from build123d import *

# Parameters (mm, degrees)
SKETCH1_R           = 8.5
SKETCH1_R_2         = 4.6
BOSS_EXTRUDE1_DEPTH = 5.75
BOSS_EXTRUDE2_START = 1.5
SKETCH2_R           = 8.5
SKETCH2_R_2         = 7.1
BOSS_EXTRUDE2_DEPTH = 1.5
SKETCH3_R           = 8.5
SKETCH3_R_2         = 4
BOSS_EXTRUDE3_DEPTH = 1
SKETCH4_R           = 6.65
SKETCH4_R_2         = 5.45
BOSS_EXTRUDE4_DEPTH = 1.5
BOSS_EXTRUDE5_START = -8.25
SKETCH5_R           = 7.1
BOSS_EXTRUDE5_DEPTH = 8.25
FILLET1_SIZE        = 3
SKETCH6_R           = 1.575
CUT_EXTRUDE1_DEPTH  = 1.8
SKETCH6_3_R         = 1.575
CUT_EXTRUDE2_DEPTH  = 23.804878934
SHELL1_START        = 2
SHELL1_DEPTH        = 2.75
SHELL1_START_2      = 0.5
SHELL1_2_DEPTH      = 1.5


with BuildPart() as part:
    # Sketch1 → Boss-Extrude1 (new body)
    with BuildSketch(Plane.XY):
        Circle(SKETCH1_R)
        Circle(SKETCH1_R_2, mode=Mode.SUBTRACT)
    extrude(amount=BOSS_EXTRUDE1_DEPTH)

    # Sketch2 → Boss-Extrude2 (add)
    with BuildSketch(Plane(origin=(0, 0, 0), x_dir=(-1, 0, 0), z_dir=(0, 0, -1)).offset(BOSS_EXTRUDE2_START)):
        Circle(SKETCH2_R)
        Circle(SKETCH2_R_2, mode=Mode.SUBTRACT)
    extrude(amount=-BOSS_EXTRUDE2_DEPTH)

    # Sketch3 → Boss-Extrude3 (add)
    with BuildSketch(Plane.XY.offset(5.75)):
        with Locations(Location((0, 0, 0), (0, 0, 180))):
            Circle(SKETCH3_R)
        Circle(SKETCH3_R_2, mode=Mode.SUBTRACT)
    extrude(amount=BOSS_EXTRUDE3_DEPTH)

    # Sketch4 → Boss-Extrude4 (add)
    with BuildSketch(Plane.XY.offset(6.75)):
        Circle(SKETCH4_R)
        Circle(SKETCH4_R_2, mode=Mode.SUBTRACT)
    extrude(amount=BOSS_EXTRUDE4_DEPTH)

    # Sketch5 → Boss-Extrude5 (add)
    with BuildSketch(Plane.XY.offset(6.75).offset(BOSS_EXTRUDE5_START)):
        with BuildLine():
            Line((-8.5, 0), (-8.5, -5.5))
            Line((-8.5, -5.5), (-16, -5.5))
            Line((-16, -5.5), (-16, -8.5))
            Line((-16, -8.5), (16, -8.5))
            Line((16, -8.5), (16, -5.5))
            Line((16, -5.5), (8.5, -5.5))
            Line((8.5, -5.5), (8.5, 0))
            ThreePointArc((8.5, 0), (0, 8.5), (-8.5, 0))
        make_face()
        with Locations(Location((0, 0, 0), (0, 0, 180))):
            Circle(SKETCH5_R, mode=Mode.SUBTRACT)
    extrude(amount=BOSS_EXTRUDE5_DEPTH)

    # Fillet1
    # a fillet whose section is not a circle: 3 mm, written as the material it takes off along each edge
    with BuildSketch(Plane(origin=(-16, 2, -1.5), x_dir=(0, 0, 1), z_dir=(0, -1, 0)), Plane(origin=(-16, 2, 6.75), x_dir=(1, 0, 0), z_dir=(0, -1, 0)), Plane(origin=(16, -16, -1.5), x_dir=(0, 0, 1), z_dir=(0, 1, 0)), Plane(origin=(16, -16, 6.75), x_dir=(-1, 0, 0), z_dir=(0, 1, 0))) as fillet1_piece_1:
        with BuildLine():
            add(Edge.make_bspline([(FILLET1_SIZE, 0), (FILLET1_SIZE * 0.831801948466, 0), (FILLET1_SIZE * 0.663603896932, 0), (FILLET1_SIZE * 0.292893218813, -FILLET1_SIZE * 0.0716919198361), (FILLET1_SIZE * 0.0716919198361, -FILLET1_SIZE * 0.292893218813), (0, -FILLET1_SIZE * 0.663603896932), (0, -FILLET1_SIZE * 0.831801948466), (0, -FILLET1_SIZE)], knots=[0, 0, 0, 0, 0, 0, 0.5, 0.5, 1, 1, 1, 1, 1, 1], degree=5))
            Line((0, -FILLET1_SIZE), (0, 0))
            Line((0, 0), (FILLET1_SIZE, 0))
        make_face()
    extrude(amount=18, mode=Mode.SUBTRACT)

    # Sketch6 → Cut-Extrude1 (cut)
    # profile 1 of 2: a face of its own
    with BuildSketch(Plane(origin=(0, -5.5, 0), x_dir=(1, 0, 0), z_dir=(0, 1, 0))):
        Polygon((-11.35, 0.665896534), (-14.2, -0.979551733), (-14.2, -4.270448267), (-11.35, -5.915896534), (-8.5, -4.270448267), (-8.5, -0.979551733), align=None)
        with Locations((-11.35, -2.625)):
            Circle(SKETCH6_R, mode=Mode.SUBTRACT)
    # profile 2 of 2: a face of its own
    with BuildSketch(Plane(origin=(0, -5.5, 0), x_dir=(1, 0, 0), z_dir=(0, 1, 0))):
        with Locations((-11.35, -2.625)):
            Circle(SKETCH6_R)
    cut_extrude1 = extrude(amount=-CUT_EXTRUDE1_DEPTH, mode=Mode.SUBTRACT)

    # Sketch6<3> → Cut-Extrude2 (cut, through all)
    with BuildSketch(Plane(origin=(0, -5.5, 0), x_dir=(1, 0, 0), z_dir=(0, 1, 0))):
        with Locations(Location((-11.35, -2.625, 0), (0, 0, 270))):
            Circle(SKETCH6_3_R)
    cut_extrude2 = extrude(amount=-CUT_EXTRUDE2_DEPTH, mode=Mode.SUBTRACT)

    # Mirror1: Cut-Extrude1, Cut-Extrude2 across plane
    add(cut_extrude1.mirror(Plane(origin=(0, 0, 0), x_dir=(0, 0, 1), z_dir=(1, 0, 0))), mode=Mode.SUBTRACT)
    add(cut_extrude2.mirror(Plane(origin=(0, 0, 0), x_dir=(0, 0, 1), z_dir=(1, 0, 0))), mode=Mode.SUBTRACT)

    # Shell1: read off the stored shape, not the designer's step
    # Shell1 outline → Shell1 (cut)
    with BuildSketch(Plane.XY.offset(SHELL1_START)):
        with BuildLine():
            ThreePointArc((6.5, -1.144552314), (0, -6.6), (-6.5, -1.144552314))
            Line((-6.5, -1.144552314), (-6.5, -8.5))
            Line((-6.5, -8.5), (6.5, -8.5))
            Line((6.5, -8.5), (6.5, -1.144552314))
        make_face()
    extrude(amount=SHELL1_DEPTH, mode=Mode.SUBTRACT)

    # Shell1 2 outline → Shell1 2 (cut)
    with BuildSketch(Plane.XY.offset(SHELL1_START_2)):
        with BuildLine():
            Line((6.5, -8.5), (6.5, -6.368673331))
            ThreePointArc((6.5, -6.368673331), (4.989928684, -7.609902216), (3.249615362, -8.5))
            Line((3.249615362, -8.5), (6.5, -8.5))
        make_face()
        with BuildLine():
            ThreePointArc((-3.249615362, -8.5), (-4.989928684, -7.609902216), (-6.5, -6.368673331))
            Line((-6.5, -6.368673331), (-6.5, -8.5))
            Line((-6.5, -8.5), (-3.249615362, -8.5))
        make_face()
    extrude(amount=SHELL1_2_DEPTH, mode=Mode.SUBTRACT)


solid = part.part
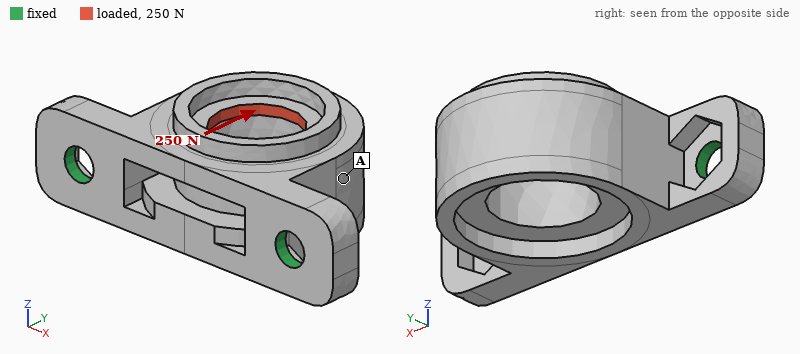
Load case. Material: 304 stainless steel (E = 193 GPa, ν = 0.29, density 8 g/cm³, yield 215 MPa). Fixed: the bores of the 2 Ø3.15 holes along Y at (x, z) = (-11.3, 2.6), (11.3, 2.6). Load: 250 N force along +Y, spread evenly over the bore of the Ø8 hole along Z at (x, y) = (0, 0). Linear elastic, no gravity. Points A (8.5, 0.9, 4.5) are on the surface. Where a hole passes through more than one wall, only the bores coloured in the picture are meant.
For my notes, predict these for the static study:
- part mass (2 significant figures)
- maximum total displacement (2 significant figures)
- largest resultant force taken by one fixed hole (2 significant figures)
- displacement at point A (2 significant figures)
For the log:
13 g
13 µm
150 N
7.1 µm
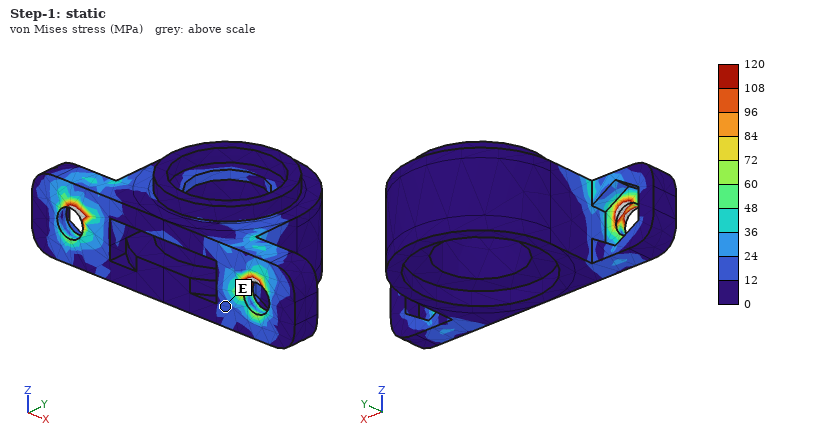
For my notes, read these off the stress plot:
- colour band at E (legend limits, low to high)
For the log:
12 to 24 MPa
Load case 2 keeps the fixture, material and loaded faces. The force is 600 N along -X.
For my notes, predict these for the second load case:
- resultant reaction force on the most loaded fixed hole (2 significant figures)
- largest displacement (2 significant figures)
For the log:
390 N
6.0 µm
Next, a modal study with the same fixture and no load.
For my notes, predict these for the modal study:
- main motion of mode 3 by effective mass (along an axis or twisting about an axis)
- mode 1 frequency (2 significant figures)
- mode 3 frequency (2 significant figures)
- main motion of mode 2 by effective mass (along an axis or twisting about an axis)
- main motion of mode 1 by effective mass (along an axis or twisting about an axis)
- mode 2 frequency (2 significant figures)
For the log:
along Y
5600 Hz
22 kHz
along X
along Z
18 kHz
